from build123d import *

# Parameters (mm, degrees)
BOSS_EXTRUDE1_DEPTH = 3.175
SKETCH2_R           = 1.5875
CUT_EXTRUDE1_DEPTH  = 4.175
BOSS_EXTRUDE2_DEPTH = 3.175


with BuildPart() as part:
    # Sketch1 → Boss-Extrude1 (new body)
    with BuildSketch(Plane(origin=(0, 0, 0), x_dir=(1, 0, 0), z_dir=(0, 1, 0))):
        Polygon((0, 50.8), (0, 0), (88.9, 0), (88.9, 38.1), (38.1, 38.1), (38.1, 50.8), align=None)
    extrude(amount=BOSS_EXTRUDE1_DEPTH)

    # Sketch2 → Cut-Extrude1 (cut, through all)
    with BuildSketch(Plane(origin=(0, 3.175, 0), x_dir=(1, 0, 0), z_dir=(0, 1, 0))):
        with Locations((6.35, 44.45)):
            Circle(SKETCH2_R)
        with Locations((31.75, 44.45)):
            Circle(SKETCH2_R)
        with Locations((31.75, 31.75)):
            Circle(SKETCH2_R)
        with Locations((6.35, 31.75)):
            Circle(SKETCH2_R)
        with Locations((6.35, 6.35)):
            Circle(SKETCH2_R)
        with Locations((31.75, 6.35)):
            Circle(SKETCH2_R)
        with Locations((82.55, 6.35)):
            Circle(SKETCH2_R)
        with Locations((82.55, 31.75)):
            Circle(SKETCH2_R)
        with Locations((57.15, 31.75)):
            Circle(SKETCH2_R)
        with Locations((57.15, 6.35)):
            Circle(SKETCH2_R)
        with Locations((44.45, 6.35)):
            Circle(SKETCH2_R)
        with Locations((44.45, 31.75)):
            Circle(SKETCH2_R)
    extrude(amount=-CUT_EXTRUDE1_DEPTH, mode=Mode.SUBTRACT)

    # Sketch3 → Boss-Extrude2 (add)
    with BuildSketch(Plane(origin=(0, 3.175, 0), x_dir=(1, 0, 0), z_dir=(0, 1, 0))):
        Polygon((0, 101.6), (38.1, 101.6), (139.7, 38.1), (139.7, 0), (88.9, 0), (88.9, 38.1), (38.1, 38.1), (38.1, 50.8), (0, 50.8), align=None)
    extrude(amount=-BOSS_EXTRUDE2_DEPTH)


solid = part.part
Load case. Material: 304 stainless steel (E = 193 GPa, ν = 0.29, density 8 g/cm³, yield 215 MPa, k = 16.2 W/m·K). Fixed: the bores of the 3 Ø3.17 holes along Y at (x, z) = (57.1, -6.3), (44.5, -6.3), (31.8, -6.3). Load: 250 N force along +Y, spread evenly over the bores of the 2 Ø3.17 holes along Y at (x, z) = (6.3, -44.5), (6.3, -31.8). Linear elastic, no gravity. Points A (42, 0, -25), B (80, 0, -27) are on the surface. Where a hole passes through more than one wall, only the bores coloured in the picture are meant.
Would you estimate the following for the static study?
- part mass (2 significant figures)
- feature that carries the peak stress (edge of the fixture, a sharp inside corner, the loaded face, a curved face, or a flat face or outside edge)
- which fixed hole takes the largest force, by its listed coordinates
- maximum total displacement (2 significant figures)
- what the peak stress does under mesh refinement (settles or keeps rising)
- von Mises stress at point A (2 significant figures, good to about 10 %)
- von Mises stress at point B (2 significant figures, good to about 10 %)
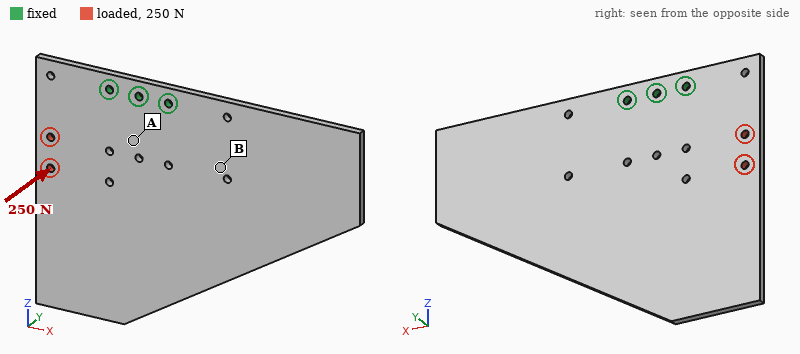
280 g
edge of the fixture
(31.8, -6.3)
0.51 mm
keeps rising
56 MPa
15 MPa
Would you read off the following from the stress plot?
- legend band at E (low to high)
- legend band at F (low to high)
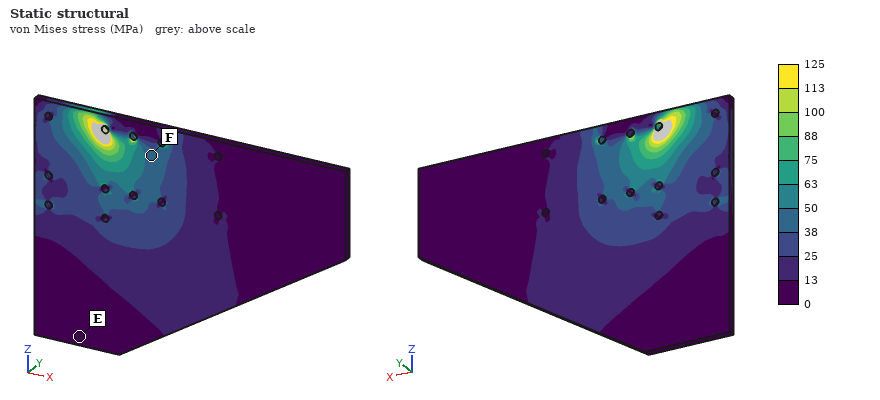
0 to 13 MPa
38 to 50 MPa
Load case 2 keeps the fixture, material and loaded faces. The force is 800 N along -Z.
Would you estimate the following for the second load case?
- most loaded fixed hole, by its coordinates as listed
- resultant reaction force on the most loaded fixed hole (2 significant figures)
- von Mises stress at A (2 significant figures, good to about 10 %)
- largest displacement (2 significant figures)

(31.8, -6.3)
1.4 kN
10 MPa
20 µm
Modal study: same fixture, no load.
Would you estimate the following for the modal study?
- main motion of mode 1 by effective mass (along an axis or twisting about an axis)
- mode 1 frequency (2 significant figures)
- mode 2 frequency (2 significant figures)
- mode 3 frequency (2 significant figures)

along Y
290 Hz
340 Hz
790 Hz
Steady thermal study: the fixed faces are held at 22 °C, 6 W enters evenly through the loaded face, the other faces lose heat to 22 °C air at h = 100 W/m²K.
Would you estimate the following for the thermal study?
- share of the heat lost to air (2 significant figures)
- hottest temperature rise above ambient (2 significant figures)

95 %
40 K
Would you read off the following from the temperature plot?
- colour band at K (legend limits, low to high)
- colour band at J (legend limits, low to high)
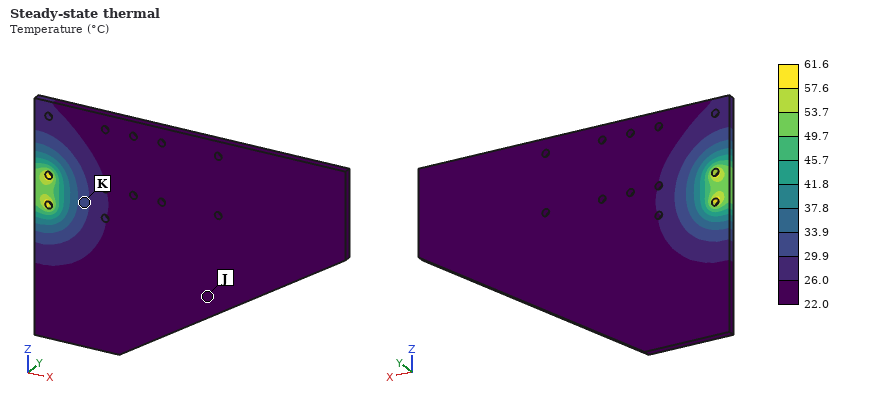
29.9 to 33.9 °C
22.0 to 26.0 °C
